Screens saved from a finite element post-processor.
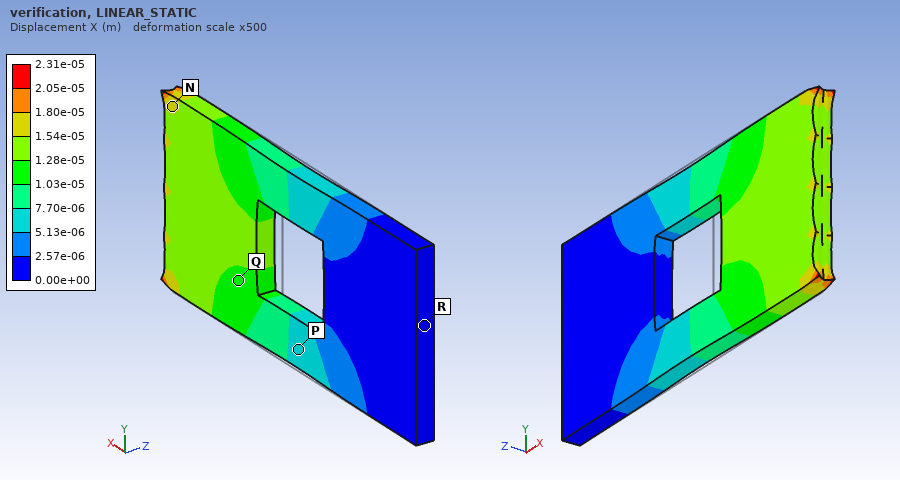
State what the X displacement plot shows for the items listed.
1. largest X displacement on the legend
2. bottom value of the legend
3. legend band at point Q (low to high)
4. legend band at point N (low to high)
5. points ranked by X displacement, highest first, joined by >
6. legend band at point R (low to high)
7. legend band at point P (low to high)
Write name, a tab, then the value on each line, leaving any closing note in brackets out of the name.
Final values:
largest X displacement on the legend	2.31e-05 m
bottom value of the legend	0.00e+00 m
legend band at point Q	1.03e-05 to 1.28e-05 m
legend band at point N	1.54e-05 to 1.80e-05 m
points ranked by X displacement, highest first, joined by >	N > Q > P > R
legend band at point R	0.00e+00 to 2.57e-06 m
legend band at point P	5.13e-06 to 7.70e-06 m
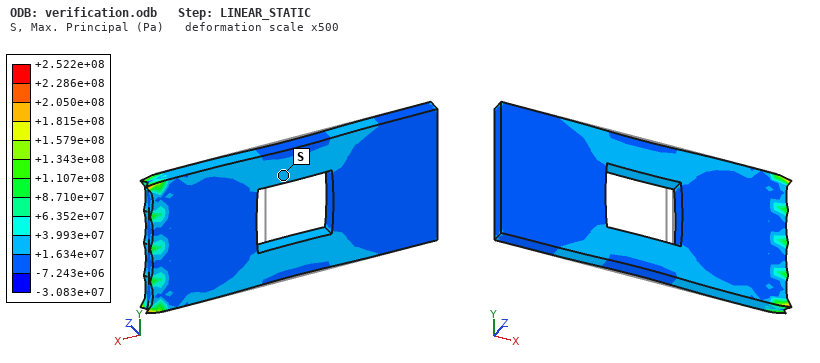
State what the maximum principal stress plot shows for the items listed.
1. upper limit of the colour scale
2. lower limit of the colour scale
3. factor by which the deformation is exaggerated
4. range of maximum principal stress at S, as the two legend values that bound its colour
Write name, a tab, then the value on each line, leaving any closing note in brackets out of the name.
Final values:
upper limit of the colour scale	+2.522e+08 Pa
lower limit of the colour scale	-3.083e+07 Pa
factor by which the deformation is exaggerated	500
range of maximum principal stress at S, as the two legend values that bound its colour	+1.634e+07 to +3.993e+07 Pa
